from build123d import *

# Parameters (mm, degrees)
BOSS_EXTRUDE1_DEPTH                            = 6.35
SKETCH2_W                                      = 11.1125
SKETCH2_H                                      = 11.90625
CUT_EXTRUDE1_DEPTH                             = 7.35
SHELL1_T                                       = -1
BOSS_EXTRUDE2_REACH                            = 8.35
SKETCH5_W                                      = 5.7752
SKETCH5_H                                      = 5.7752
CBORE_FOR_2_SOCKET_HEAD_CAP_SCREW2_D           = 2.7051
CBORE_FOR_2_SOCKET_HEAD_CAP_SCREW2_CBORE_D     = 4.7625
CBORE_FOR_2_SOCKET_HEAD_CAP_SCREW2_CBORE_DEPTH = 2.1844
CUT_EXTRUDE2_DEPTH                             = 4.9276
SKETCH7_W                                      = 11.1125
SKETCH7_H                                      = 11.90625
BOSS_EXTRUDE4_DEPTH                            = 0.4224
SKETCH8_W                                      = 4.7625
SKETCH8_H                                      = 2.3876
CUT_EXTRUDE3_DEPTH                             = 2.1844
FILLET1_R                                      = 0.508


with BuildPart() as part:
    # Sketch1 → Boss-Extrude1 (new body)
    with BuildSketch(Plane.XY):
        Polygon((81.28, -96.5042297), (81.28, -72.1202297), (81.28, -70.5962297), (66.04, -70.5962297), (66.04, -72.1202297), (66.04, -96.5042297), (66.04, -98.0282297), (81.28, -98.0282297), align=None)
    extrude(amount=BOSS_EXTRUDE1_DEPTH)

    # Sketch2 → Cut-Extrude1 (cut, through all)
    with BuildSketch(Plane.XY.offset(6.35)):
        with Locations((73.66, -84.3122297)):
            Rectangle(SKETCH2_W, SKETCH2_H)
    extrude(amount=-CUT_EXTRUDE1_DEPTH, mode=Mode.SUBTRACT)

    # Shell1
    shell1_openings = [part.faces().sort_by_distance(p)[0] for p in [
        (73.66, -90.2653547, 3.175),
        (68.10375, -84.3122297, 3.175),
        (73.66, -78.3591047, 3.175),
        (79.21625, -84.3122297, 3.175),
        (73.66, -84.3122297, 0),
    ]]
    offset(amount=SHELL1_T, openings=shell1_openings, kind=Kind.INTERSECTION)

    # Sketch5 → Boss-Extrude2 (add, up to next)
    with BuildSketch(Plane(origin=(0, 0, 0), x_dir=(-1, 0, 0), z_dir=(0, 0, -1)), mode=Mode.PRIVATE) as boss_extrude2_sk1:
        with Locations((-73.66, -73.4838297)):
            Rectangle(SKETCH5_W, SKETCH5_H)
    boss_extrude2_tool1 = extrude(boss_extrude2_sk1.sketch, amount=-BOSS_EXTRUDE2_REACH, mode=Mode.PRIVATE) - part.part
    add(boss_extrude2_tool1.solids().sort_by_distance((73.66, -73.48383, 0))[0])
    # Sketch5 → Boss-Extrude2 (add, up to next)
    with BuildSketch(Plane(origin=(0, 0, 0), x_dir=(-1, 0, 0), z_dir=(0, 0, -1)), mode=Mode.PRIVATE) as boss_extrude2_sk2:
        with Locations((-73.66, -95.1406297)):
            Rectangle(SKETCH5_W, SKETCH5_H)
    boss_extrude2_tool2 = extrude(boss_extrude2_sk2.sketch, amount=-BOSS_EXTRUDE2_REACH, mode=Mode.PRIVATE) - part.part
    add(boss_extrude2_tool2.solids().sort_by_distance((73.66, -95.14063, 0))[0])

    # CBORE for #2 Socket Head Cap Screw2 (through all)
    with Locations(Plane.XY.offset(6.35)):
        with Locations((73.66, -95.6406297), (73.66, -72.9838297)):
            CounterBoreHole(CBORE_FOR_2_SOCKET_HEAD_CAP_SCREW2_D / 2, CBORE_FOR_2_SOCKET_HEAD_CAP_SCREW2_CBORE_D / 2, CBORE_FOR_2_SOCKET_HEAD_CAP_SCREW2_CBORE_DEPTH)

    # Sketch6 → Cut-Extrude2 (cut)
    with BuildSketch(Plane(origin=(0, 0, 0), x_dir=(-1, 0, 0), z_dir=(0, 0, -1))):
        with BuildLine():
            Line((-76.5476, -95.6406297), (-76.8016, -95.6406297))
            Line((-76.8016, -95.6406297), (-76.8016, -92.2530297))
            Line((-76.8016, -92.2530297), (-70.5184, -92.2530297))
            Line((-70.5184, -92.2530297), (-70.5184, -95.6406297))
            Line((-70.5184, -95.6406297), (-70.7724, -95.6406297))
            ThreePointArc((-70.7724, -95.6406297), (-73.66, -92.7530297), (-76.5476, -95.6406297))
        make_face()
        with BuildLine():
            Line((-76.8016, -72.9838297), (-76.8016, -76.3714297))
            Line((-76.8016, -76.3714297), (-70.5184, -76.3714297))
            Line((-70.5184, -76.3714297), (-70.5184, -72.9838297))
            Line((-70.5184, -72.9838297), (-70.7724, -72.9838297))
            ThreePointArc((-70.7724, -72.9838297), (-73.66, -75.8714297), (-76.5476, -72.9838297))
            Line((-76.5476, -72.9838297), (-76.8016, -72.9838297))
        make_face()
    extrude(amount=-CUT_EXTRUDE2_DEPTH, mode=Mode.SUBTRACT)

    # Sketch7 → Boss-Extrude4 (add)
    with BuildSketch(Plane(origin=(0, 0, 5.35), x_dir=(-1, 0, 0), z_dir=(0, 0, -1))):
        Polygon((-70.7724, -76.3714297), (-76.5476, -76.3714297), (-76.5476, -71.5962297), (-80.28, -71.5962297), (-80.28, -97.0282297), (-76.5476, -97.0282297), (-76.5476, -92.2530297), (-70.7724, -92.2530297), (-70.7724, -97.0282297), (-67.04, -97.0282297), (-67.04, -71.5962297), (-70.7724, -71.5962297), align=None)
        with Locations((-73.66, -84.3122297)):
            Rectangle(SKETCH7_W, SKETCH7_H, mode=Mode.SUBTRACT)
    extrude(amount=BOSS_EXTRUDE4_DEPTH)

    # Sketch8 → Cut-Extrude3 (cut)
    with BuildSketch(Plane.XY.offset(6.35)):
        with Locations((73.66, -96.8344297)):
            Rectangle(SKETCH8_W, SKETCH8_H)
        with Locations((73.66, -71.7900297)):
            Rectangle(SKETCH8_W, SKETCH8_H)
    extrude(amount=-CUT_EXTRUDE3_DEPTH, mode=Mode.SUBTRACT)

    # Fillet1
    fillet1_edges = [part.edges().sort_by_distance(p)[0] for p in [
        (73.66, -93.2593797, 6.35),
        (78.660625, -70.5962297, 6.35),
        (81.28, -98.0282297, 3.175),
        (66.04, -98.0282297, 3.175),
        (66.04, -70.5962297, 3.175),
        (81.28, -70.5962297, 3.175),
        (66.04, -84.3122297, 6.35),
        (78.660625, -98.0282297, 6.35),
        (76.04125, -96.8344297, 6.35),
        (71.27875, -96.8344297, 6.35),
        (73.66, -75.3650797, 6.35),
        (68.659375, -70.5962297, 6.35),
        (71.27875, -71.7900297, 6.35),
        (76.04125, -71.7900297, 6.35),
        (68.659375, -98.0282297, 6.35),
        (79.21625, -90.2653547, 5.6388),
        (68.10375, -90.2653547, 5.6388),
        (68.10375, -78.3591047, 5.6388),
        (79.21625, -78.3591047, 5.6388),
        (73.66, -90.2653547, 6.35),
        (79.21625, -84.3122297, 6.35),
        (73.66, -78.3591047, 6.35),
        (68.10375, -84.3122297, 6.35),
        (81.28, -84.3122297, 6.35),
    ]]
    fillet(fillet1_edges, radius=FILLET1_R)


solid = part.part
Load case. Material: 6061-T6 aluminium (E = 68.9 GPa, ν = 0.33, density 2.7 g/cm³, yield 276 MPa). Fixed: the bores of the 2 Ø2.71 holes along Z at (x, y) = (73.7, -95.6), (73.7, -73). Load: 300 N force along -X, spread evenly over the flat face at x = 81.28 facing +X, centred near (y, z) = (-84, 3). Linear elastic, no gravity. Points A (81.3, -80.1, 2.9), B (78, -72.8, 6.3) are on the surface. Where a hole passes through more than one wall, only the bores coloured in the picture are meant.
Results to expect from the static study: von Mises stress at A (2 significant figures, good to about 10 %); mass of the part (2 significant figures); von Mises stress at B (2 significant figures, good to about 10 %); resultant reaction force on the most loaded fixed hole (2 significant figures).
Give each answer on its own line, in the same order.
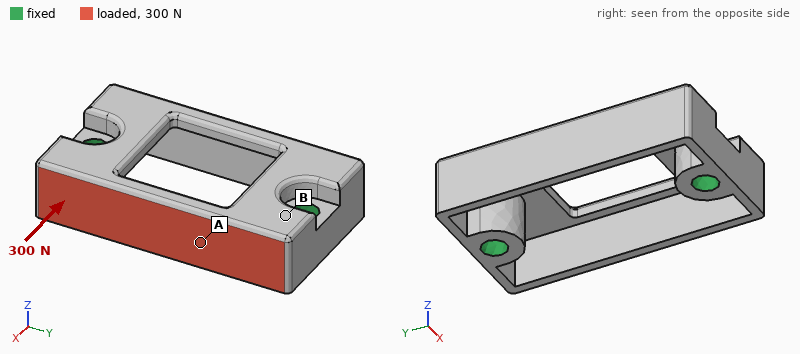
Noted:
55 MPa
2.3 g
23 MPa
160 N
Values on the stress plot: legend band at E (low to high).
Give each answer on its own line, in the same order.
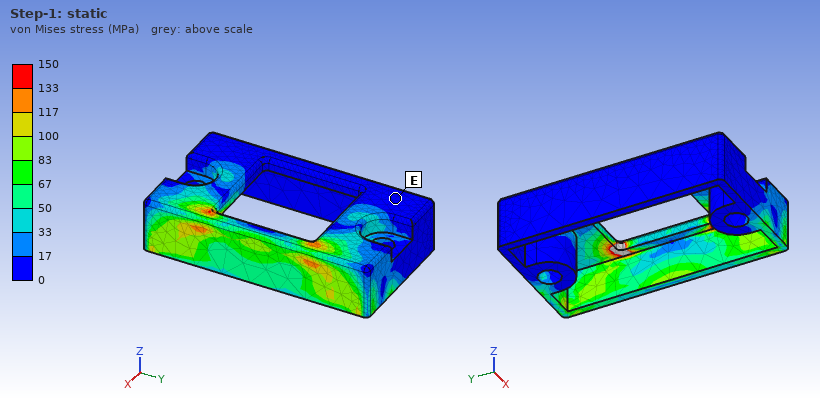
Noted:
0 to 17 MPa
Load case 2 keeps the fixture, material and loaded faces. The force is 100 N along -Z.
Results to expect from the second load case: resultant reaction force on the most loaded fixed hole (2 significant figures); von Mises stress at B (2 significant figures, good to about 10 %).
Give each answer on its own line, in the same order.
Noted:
54 N
11 MPa
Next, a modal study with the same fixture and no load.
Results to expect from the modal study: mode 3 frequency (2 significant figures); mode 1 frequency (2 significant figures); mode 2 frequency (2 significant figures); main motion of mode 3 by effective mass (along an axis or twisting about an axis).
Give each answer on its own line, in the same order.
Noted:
19 kHz
15 kHz
15 kHz
along X
